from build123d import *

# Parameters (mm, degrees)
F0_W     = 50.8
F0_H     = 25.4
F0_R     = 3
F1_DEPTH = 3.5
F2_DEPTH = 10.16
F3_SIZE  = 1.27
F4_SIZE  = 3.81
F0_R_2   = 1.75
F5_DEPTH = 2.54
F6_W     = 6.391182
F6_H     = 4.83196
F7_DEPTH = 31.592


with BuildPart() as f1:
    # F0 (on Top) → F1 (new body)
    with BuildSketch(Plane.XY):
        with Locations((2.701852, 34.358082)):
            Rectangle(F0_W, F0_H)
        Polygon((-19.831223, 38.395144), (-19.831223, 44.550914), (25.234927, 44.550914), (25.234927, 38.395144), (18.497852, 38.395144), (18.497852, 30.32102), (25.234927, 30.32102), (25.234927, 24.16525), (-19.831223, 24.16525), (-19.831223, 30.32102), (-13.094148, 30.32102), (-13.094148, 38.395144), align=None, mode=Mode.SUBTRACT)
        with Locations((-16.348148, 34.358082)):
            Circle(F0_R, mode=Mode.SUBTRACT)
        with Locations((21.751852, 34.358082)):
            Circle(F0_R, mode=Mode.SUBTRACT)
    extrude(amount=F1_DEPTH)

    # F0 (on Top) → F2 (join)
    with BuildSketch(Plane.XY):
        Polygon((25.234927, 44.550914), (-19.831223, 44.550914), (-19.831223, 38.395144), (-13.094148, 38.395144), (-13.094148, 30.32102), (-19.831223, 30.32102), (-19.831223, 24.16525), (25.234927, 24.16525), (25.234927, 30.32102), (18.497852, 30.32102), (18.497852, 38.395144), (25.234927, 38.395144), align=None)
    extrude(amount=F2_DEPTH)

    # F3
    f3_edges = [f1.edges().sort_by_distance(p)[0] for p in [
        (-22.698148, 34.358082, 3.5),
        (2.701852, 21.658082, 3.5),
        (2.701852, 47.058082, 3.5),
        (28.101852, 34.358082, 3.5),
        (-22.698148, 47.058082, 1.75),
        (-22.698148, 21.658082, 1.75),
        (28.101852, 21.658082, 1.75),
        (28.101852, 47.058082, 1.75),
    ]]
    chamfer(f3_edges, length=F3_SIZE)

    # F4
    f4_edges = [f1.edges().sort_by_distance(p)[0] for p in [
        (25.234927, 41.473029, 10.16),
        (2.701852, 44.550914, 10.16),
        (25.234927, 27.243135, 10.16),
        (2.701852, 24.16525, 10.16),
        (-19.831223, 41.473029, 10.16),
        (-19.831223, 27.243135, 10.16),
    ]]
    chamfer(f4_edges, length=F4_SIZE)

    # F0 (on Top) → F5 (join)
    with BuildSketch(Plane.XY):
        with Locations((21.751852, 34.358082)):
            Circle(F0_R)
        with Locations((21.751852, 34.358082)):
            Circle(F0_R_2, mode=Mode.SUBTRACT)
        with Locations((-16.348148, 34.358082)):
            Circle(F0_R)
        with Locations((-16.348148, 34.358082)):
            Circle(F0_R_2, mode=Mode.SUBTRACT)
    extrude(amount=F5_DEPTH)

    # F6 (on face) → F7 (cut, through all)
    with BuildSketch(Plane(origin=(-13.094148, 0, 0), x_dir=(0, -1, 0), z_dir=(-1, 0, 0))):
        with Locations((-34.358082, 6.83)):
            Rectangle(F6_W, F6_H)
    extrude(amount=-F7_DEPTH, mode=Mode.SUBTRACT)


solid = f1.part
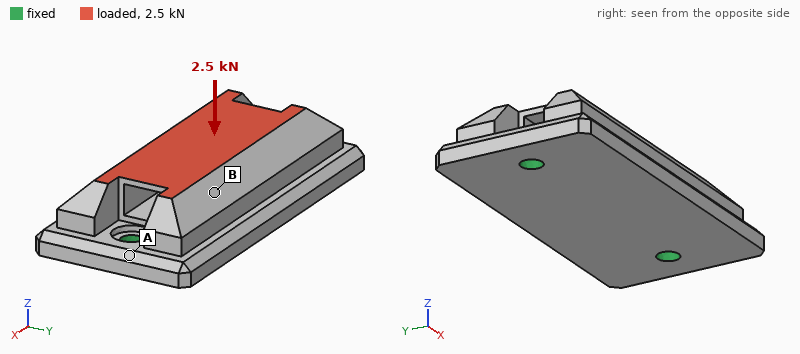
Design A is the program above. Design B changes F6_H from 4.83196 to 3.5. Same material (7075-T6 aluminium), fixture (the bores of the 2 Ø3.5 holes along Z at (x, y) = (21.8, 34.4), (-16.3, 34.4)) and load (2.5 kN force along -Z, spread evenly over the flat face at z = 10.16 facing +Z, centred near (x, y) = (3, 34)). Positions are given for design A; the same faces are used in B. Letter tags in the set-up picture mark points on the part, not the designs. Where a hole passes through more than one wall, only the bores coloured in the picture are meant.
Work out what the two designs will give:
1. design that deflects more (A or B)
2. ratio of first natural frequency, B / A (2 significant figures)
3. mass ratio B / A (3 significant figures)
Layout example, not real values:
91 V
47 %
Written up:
A
1.0
1.03
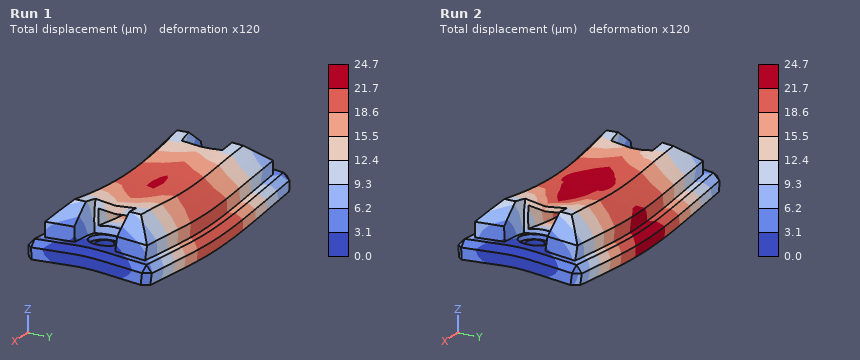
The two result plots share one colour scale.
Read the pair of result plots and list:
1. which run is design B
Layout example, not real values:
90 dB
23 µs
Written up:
Run 1
